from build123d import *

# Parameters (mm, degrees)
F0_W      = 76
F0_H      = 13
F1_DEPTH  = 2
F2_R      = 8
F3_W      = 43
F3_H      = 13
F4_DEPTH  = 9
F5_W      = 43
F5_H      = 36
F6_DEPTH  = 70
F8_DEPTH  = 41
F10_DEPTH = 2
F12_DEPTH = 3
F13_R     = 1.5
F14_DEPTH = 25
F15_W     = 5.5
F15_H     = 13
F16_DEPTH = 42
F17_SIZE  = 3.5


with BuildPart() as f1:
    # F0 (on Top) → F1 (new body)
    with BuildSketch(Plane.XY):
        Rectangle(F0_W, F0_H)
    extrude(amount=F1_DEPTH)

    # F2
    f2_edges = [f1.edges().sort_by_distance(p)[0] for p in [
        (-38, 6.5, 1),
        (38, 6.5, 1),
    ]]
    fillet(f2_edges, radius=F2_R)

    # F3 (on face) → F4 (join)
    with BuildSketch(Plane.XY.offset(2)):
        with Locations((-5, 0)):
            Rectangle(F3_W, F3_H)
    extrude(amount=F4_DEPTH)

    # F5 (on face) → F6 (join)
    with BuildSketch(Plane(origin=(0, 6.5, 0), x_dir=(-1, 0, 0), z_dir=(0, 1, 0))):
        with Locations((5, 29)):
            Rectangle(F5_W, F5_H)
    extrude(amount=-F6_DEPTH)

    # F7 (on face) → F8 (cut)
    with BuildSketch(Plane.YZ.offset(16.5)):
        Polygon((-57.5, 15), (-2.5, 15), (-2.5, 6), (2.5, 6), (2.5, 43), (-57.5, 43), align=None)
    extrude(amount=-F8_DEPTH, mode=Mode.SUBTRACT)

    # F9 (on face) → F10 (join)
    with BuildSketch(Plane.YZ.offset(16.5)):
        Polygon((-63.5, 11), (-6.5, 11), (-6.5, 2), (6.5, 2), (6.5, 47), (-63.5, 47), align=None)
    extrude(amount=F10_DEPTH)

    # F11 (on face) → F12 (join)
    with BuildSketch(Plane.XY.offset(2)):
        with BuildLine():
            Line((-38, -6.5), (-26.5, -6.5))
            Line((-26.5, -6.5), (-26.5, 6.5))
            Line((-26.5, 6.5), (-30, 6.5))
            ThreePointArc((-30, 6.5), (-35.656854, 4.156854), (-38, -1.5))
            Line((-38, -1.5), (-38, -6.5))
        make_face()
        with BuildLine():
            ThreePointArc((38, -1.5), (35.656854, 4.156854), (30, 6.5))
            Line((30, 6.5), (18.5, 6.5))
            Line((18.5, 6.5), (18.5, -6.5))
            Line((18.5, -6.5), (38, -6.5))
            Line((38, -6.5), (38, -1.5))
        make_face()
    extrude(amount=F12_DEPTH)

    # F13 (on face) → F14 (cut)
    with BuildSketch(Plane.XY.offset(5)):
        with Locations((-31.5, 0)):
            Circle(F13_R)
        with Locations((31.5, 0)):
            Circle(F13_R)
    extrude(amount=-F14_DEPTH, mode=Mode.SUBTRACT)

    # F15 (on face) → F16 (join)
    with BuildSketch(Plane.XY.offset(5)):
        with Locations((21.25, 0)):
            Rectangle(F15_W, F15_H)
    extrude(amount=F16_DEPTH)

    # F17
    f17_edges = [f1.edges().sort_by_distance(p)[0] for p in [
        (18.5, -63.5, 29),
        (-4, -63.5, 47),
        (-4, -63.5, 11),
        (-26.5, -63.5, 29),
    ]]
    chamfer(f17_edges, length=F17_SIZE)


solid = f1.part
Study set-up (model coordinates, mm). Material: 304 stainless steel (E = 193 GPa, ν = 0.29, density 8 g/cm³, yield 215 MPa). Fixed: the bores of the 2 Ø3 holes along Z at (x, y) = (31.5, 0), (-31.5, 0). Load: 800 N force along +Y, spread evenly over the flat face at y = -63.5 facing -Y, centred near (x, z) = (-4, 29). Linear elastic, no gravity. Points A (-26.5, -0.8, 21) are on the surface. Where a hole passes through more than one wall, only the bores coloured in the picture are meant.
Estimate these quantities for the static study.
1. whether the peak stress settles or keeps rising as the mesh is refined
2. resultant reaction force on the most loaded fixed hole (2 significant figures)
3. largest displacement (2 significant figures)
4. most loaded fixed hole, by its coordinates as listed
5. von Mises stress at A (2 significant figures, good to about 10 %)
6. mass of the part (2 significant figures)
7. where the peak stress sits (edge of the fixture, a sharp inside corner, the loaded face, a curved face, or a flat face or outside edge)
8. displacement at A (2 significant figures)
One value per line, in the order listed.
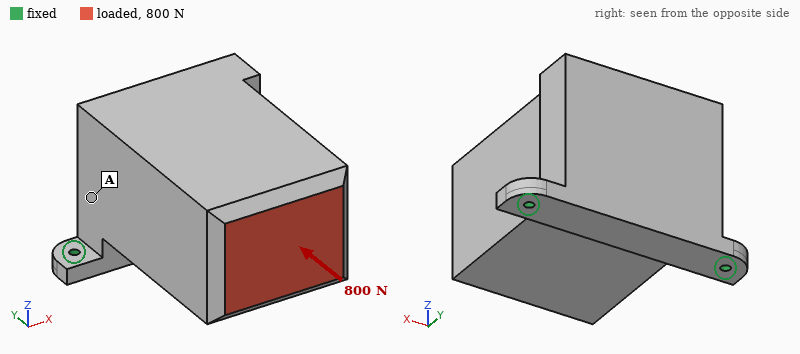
keeps rising
450 N
0.21 mm
(-31.5, 0)
21 MPa
420 g
edge of the fixture
0.050 mm
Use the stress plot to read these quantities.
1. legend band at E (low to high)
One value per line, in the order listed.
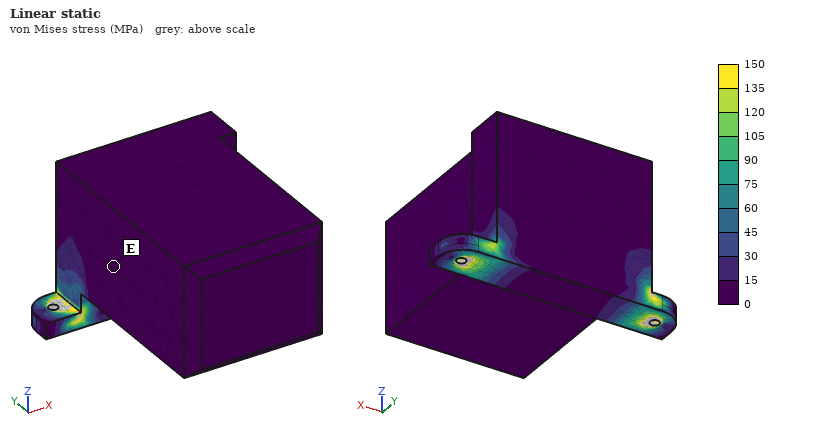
0 to 15 MPa
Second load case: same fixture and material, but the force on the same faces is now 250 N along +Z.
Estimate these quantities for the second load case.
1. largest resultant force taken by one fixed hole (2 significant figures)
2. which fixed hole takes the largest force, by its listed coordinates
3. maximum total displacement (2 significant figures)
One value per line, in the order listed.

140 N
(-31.5, 0)
0.17 mm
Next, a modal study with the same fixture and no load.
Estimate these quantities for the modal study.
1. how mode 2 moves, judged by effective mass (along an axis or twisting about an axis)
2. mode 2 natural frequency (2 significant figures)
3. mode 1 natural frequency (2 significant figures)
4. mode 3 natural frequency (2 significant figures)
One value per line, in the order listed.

along X
1900 Hz
480 Hz
3500 Hz
